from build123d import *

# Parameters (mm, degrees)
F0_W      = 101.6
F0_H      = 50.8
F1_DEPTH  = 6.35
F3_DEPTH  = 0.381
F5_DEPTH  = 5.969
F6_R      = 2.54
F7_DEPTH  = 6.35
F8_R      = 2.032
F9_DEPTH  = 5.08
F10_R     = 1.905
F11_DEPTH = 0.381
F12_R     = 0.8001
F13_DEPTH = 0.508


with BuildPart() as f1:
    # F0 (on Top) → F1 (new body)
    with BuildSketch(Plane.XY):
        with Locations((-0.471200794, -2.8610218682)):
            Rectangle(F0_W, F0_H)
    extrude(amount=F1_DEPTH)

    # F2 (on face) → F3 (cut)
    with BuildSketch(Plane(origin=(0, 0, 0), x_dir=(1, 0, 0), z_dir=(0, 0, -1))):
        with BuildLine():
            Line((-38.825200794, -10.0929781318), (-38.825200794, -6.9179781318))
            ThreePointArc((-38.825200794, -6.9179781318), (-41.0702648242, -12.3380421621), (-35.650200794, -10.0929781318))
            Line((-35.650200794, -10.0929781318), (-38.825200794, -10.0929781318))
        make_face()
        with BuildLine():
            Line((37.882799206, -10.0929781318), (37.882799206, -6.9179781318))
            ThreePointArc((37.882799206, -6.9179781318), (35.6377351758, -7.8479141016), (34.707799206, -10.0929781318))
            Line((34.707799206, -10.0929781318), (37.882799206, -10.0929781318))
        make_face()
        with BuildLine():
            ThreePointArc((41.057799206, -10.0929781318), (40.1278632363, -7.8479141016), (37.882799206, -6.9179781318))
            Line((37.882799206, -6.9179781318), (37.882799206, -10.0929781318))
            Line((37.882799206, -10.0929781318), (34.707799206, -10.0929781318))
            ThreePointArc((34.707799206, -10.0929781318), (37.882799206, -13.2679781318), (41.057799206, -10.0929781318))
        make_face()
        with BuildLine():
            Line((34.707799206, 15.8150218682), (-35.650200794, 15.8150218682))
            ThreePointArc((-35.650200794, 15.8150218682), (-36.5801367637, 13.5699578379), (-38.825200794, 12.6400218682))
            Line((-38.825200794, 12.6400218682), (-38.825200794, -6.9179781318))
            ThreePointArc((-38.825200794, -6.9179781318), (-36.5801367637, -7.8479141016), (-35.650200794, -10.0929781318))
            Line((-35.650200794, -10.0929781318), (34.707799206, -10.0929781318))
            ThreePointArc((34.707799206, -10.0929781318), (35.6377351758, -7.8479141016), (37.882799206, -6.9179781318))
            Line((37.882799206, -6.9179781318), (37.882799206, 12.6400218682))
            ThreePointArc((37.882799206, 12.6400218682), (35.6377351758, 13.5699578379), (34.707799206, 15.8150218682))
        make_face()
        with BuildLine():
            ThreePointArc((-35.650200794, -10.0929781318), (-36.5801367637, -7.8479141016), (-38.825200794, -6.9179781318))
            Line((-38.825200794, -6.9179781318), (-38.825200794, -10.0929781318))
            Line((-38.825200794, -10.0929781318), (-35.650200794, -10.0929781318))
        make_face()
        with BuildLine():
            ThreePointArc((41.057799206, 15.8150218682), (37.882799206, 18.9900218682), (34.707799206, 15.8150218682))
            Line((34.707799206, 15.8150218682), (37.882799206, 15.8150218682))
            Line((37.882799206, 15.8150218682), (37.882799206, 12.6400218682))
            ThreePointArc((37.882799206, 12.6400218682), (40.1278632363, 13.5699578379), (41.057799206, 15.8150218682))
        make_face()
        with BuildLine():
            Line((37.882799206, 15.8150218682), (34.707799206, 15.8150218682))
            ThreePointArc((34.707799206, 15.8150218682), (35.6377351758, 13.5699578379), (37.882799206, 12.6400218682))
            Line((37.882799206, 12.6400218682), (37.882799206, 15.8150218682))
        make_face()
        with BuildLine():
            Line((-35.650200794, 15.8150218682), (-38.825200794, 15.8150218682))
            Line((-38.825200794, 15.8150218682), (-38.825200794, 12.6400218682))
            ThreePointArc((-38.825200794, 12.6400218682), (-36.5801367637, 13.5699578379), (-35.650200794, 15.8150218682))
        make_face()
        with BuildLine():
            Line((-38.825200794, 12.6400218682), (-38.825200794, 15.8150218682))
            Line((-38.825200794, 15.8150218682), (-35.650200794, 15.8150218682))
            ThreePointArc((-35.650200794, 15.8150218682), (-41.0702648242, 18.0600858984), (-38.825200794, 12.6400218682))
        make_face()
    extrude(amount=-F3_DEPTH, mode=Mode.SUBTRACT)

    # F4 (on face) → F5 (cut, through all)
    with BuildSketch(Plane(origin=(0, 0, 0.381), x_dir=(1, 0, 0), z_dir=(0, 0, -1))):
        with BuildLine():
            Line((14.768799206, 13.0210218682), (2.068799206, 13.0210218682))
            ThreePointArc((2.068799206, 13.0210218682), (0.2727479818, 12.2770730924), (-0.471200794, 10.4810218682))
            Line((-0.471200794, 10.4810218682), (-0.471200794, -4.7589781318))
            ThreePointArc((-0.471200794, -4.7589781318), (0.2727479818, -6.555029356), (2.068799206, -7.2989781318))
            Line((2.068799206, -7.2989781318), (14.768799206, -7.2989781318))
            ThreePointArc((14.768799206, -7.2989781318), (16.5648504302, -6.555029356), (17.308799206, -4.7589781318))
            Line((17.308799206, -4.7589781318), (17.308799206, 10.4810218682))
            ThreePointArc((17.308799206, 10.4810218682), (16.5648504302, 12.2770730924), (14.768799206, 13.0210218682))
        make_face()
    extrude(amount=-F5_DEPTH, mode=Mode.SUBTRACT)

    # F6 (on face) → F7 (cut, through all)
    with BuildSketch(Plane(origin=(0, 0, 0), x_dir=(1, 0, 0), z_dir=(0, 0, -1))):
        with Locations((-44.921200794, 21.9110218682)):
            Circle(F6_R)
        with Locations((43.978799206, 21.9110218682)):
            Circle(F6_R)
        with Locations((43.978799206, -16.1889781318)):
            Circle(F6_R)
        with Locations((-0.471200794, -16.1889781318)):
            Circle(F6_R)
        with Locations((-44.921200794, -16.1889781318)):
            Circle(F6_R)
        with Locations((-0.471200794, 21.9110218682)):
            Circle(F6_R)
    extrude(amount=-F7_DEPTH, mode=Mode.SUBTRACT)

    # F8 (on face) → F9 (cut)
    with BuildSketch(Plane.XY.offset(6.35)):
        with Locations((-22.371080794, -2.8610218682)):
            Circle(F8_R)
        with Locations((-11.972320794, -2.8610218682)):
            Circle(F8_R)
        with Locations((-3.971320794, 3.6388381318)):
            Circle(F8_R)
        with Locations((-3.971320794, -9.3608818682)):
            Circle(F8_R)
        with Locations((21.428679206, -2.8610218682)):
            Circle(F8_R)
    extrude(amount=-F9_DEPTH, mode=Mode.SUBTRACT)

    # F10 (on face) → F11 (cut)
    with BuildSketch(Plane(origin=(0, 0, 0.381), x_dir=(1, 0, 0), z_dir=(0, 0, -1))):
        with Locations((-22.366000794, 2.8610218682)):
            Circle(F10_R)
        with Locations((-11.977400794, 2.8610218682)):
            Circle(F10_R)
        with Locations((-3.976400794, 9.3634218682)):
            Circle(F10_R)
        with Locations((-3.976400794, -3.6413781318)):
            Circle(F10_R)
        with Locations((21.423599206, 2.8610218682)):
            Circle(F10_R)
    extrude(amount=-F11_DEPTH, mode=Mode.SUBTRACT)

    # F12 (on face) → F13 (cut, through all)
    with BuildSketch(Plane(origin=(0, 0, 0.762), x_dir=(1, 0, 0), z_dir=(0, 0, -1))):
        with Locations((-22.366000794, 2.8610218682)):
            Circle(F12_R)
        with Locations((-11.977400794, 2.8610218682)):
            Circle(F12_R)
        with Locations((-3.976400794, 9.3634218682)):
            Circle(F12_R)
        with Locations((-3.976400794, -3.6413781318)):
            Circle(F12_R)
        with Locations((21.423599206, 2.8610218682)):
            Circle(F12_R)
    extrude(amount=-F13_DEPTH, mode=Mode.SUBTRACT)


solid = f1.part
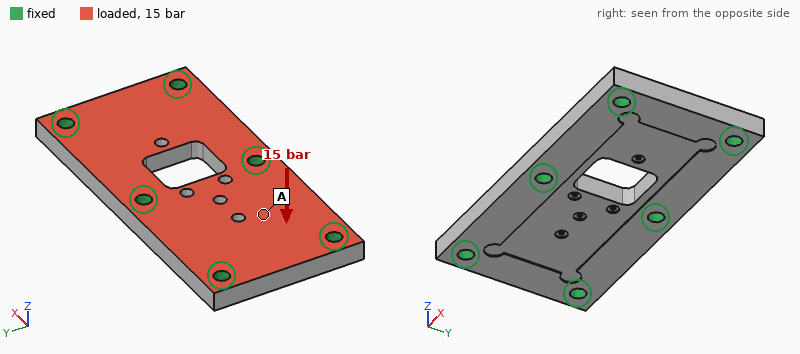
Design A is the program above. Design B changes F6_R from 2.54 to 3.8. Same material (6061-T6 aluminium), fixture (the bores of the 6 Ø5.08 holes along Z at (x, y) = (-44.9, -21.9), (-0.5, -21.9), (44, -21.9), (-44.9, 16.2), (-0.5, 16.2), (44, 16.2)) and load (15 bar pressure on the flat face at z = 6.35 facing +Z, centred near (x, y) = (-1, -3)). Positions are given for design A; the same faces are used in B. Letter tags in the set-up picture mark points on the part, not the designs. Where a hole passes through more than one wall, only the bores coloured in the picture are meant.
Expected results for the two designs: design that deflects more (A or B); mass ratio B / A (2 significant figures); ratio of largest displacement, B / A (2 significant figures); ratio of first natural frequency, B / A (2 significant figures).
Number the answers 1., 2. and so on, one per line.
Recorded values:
1. A
2. 0.97
3. 0.82
4. 1.1
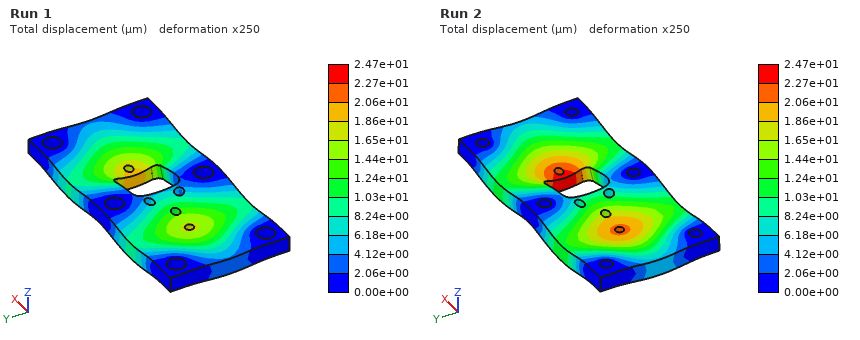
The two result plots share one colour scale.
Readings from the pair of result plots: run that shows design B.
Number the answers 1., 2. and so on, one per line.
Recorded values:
1. Run 1
